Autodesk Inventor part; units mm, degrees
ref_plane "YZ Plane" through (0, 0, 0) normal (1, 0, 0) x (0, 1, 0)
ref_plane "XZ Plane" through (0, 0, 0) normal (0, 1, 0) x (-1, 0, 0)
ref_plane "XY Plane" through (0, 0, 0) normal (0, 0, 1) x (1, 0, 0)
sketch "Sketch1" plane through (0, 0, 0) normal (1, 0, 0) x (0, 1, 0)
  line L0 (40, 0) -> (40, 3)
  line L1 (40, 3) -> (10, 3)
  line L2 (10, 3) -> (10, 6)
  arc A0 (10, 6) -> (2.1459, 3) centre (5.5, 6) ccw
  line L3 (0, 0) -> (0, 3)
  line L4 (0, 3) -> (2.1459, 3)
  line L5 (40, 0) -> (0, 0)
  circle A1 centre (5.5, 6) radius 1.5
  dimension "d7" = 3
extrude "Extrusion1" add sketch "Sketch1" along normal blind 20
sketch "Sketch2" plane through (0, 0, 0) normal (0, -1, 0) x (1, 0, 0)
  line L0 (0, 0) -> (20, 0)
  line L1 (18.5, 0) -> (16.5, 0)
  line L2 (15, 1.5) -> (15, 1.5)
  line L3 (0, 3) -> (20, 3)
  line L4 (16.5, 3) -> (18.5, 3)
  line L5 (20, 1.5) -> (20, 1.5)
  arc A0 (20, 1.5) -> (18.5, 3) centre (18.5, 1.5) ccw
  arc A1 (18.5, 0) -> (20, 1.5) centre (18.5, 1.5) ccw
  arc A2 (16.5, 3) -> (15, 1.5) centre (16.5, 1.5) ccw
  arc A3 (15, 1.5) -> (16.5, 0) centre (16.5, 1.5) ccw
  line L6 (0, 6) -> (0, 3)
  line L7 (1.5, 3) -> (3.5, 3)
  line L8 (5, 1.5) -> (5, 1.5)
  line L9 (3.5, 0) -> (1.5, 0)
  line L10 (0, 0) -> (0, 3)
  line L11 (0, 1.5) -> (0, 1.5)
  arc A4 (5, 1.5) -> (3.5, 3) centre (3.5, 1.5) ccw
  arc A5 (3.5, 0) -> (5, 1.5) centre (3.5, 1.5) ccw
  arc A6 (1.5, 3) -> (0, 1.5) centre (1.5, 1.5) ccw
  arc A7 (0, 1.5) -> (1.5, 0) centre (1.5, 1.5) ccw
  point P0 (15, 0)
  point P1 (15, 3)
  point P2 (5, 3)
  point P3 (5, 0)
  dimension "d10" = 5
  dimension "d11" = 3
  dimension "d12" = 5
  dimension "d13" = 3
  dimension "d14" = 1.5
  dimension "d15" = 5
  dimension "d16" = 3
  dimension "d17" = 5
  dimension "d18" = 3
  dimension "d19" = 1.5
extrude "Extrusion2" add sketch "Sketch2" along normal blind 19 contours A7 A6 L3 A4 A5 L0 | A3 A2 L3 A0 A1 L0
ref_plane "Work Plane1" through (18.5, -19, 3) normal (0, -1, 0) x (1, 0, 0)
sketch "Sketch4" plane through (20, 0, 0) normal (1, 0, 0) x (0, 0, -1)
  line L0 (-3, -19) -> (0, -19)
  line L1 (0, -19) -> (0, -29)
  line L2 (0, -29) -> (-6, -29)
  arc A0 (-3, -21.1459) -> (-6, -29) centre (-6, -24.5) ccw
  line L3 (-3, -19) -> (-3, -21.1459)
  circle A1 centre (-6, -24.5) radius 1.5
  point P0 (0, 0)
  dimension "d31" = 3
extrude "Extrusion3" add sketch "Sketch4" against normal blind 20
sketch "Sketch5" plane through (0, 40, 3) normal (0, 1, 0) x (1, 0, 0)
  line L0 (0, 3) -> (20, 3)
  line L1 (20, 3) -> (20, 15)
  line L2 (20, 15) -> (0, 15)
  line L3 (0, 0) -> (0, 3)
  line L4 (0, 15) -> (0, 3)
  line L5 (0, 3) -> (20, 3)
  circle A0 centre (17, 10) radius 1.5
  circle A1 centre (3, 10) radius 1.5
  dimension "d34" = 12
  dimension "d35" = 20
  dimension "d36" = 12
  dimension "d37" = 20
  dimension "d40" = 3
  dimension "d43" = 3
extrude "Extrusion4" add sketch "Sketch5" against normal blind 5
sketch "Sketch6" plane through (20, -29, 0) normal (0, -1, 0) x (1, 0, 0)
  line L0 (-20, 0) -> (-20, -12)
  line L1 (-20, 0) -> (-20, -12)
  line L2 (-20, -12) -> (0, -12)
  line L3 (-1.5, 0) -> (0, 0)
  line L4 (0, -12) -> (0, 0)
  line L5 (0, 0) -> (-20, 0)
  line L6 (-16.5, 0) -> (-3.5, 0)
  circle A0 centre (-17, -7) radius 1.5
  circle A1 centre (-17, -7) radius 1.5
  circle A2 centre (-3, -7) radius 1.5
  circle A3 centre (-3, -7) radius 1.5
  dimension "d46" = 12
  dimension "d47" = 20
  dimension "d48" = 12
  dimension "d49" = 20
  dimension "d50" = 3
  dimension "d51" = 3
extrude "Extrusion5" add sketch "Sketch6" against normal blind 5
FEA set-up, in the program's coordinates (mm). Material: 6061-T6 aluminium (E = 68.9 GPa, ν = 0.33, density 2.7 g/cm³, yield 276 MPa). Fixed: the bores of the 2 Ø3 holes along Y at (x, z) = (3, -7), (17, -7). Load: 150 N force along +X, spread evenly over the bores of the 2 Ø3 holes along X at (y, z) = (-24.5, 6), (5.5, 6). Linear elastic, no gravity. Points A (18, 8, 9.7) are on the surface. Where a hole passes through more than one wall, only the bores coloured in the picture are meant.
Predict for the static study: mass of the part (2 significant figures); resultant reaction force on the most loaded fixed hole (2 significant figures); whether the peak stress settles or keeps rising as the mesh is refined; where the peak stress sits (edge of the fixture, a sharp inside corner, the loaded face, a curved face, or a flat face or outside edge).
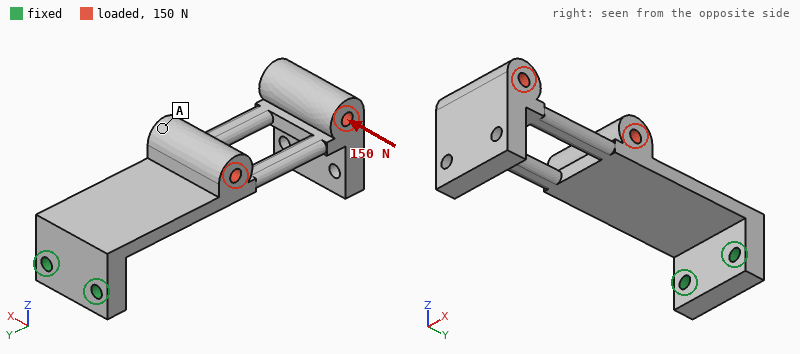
21 g
480 N
keeps rising
edge of the fixture
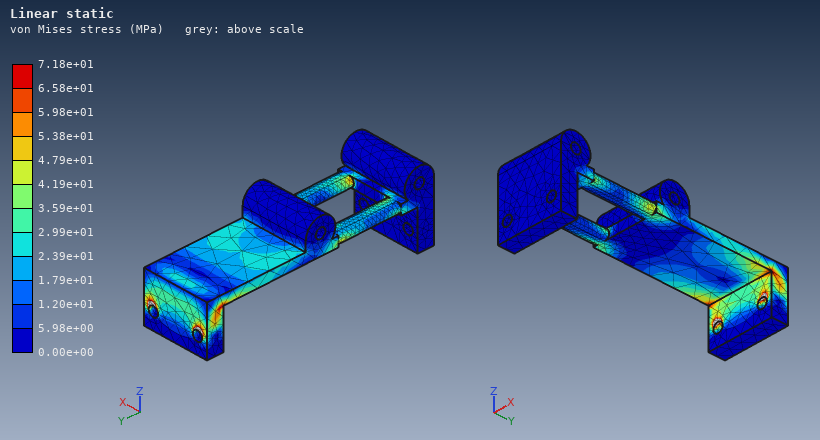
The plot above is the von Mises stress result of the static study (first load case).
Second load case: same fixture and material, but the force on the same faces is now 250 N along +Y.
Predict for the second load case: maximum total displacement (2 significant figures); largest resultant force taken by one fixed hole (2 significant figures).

0.86 mm
130 N
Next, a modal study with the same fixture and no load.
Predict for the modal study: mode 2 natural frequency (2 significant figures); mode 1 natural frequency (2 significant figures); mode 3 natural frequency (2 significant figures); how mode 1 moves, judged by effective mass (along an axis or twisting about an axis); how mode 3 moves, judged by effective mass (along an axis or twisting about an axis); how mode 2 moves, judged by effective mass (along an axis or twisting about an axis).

1300 Hz
320 Hz
1700 Hz
along Z
along Z
along X
